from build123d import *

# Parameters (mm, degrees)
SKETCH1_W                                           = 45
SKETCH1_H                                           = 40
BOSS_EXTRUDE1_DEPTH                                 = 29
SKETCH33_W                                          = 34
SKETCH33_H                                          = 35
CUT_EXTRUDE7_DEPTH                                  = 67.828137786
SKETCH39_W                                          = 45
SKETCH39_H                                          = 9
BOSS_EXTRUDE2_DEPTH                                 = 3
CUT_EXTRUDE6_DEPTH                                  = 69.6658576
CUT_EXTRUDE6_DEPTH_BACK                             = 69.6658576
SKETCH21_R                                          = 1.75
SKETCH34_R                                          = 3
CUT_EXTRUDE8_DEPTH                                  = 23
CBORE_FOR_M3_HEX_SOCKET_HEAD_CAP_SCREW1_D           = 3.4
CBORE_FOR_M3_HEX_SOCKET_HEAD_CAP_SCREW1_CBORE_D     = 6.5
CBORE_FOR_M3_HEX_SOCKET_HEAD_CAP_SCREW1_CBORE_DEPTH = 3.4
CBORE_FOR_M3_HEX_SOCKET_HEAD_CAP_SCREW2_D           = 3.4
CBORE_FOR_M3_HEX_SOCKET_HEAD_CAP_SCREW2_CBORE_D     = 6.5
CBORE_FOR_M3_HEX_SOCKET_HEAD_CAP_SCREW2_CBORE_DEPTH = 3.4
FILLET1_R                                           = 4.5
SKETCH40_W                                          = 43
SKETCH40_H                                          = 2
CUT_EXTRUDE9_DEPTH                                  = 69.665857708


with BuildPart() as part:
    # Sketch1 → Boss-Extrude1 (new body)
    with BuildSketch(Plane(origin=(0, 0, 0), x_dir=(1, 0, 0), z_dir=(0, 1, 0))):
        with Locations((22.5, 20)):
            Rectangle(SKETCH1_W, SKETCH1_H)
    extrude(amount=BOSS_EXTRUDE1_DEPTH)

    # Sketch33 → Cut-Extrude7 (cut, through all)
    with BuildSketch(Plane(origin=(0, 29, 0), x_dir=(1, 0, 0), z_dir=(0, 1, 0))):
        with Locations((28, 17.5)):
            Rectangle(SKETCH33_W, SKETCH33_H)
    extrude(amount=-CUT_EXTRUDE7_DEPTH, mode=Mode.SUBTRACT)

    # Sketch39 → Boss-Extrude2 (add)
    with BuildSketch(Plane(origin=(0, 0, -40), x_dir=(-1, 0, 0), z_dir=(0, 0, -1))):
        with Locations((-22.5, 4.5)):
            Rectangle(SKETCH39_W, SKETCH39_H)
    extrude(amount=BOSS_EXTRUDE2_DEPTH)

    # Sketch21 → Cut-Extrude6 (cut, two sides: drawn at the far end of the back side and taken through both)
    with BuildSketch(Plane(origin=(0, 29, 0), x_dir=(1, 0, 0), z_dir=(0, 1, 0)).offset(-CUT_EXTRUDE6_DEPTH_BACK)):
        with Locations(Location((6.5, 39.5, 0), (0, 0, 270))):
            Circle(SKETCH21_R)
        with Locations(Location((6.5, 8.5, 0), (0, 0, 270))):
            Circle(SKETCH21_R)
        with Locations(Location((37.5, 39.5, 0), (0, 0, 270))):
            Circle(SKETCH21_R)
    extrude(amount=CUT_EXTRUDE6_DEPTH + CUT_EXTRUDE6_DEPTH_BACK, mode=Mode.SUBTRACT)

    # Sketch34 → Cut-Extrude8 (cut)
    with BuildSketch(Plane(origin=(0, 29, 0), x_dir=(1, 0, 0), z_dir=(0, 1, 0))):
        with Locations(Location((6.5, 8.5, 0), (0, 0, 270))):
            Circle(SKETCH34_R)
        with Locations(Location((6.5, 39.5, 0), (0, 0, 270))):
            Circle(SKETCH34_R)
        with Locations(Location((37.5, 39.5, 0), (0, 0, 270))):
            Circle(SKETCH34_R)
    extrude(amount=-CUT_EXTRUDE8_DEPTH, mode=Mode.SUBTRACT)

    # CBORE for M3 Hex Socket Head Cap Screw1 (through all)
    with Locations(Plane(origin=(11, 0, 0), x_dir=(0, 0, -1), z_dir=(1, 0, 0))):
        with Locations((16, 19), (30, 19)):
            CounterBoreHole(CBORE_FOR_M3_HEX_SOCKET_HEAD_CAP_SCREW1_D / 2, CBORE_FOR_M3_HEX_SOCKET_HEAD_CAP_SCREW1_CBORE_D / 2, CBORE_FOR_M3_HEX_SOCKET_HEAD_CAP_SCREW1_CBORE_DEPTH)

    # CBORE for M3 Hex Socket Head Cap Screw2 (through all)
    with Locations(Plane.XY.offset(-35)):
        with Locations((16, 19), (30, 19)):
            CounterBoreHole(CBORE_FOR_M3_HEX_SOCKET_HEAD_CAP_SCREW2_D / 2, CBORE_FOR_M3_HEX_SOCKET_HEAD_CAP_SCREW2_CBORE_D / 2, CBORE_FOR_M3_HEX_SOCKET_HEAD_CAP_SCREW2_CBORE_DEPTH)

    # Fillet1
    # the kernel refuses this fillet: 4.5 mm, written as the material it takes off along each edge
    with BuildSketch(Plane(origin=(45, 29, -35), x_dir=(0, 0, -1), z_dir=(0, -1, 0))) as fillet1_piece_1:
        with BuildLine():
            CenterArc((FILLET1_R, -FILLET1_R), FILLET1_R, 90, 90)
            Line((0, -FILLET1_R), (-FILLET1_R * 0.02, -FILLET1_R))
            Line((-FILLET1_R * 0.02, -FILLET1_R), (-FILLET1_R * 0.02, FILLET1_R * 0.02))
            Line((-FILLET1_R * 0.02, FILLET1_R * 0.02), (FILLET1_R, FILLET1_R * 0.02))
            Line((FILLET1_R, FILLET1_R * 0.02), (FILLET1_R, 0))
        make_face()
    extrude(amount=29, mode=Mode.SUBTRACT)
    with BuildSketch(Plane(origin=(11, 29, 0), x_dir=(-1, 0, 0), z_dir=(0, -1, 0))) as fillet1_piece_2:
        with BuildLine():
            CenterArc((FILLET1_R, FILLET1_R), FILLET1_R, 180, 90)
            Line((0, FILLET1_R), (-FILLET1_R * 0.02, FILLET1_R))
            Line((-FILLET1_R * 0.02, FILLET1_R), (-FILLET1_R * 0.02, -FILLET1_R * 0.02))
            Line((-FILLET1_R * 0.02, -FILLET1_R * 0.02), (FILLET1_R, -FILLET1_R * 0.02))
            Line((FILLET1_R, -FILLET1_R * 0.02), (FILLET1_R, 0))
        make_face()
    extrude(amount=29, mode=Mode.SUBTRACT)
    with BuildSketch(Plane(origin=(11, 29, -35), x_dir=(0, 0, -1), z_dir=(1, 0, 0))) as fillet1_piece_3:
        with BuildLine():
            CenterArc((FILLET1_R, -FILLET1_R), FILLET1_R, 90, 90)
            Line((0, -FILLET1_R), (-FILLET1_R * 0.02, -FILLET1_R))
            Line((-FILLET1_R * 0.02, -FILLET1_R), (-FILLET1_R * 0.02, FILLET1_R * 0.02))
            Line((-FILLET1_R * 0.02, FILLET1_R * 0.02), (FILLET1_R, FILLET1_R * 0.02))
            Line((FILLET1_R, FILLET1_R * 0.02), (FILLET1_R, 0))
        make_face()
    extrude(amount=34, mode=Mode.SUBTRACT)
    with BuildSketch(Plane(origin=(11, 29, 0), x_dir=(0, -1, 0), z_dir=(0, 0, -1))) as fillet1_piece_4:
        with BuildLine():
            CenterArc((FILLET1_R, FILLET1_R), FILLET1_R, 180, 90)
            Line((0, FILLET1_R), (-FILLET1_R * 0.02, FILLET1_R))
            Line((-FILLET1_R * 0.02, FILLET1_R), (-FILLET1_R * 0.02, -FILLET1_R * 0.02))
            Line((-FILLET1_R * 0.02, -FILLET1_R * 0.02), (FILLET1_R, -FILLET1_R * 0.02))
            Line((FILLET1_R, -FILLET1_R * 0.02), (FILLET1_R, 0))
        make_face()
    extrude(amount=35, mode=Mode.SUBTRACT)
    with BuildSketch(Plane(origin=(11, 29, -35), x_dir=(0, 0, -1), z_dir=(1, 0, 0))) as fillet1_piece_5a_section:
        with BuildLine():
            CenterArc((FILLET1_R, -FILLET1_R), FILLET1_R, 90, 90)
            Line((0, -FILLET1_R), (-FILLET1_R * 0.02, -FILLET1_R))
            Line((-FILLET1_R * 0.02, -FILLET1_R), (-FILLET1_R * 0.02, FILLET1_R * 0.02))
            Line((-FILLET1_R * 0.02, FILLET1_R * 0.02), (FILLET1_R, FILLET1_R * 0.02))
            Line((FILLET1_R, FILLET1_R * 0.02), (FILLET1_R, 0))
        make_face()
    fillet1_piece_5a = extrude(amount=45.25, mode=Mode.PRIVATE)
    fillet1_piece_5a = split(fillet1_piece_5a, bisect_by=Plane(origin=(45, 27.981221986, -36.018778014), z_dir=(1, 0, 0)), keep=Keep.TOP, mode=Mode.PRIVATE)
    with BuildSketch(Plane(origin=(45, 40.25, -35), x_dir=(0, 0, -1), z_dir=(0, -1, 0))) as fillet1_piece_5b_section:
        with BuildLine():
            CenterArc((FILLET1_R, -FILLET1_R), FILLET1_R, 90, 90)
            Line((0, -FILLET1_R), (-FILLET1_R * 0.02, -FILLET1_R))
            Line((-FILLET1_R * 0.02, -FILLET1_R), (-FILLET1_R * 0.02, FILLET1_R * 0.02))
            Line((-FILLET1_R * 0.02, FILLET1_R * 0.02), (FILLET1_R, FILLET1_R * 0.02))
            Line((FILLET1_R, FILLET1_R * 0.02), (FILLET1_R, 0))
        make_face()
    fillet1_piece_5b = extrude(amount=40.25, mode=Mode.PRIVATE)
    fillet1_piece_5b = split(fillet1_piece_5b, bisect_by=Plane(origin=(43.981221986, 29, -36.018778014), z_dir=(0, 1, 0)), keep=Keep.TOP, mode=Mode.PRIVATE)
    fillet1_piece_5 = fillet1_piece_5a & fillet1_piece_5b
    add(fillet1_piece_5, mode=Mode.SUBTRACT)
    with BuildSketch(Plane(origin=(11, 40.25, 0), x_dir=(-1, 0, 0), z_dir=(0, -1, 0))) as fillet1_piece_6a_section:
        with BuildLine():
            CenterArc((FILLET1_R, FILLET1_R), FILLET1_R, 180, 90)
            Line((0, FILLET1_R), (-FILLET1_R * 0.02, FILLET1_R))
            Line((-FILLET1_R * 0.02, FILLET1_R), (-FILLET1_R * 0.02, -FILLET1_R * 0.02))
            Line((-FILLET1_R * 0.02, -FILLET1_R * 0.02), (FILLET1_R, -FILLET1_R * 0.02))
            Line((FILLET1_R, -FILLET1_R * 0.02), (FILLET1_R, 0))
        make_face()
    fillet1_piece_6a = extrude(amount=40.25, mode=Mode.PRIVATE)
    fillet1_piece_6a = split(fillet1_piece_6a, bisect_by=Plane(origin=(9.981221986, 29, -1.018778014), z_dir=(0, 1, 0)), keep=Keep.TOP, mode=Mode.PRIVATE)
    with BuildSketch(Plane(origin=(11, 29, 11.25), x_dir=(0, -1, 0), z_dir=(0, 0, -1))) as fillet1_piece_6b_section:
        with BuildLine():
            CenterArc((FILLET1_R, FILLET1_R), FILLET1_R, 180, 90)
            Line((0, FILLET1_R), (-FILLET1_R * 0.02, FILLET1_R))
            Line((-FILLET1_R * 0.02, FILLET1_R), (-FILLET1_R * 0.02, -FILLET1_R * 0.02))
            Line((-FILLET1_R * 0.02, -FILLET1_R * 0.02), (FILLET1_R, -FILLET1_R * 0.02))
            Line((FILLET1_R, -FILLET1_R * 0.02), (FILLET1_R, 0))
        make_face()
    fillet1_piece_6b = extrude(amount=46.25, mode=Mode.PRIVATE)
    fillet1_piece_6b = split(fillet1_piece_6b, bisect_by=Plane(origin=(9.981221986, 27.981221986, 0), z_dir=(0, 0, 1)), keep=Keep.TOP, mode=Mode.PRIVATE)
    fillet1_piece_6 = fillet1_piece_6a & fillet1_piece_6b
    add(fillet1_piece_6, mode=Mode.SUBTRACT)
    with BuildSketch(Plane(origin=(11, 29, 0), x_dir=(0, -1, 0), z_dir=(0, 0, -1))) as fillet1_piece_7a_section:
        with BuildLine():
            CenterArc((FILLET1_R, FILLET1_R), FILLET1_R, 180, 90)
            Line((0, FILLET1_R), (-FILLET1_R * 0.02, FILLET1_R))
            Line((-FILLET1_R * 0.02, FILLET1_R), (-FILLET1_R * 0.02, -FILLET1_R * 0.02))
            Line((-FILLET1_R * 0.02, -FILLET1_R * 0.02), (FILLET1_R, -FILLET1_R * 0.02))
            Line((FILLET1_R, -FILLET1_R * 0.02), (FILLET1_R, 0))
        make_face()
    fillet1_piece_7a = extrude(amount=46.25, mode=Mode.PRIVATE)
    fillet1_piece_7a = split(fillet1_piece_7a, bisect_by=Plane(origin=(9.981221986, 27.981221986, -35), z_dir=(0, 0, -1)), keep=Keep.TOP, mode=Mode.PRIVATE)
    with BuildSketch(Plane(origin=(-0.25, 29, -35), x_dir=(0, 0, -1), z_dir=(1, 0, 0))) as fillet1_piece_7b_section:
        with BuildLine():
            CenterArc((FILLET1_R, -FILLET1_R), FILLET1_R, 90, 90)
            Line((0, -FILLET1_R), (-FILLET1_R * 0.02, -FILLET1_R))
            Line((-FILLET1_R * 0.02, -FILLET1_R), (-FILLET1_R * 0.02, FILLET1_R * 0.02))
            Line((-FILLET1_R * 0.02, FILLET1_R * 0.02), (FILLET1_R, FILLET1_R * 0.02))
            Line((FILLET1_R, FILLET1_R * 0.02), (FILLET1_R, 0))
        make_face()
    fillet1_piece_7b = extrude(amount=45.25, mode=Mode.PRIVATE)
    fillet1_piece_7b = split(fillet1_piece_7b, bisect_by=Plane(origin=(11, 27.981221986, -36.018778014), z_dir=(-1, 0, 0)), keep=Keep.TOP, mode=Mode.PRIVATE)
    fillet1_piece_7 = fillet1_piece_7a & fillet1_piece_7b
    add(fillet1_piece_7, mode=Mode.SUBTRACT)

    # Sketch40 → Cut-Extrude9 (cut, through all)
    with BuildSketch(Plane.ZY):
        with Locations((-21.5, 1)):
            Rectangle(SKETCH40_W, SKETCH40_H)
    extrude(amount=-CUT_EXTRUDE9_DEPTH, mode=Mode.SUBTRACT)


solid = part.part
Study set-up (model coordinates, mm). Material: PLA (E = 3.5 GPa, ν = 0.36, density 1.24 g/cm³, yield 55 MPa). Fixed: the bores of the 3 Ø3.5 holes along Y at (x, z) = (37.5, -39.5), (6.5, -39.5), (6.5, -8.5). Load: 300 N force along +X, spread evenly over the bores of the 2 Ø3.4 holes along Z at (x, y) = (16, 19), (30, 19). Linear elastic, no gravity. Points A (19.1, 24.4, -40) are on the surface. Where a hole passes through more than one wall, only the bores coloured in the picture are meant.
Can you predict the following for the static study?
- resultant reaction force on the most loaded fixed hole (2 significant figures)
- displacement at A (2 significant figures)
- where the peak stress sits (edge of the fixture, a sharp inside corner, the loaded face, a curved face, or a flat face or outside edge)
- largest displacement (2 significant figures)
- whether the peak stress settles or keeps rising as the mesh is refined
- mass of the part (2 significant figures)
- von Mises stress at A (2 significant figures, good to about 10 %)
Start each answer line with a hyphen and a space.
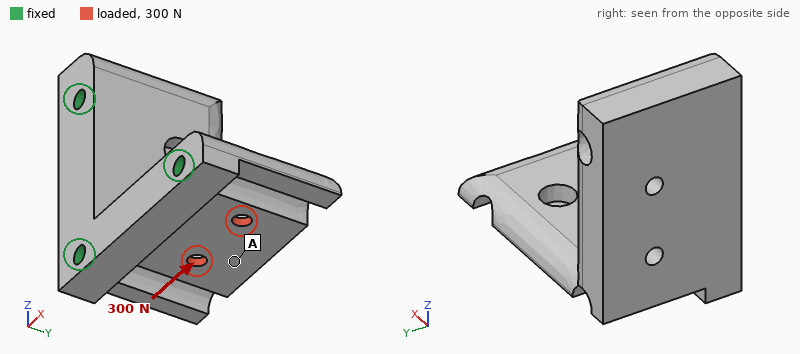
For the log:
- 200 N
- 0.053 mm
- edge of the fixture
- 0.11 mm
- keeps rising
- 18 g
- 1.8 MPa
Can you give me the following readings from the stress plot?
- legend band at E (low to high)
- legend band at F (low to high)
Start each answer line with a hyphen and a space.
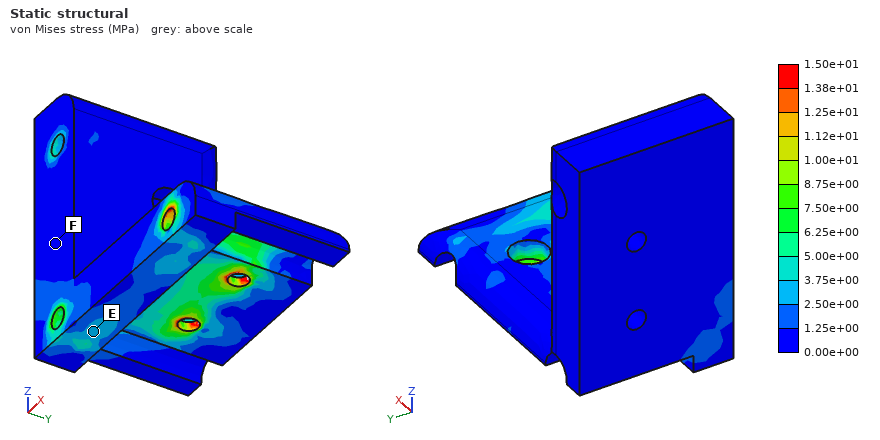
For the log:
- 2.50e+00 to 3.75e+00 MPa
- 0.00e+00 to 1.25e+00 MPa
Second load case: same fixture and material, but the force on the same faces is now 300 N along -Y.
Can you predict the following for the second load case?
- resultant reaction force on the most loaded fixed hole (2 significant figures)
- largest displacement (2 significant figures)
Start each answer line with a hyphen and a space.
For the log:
- 170 N
- 70 µm
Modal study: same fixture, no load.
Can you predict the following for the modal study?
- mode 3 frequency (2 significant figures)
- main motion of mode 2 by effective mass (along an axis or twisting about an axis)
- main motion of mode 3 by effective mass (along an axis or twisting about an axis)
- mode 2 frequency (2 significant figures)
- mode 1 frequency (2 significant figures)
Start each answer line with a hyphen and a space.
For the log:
- 5000 Hz
- along X
- along Z
- 2900 Hz
- 2600 Hz
